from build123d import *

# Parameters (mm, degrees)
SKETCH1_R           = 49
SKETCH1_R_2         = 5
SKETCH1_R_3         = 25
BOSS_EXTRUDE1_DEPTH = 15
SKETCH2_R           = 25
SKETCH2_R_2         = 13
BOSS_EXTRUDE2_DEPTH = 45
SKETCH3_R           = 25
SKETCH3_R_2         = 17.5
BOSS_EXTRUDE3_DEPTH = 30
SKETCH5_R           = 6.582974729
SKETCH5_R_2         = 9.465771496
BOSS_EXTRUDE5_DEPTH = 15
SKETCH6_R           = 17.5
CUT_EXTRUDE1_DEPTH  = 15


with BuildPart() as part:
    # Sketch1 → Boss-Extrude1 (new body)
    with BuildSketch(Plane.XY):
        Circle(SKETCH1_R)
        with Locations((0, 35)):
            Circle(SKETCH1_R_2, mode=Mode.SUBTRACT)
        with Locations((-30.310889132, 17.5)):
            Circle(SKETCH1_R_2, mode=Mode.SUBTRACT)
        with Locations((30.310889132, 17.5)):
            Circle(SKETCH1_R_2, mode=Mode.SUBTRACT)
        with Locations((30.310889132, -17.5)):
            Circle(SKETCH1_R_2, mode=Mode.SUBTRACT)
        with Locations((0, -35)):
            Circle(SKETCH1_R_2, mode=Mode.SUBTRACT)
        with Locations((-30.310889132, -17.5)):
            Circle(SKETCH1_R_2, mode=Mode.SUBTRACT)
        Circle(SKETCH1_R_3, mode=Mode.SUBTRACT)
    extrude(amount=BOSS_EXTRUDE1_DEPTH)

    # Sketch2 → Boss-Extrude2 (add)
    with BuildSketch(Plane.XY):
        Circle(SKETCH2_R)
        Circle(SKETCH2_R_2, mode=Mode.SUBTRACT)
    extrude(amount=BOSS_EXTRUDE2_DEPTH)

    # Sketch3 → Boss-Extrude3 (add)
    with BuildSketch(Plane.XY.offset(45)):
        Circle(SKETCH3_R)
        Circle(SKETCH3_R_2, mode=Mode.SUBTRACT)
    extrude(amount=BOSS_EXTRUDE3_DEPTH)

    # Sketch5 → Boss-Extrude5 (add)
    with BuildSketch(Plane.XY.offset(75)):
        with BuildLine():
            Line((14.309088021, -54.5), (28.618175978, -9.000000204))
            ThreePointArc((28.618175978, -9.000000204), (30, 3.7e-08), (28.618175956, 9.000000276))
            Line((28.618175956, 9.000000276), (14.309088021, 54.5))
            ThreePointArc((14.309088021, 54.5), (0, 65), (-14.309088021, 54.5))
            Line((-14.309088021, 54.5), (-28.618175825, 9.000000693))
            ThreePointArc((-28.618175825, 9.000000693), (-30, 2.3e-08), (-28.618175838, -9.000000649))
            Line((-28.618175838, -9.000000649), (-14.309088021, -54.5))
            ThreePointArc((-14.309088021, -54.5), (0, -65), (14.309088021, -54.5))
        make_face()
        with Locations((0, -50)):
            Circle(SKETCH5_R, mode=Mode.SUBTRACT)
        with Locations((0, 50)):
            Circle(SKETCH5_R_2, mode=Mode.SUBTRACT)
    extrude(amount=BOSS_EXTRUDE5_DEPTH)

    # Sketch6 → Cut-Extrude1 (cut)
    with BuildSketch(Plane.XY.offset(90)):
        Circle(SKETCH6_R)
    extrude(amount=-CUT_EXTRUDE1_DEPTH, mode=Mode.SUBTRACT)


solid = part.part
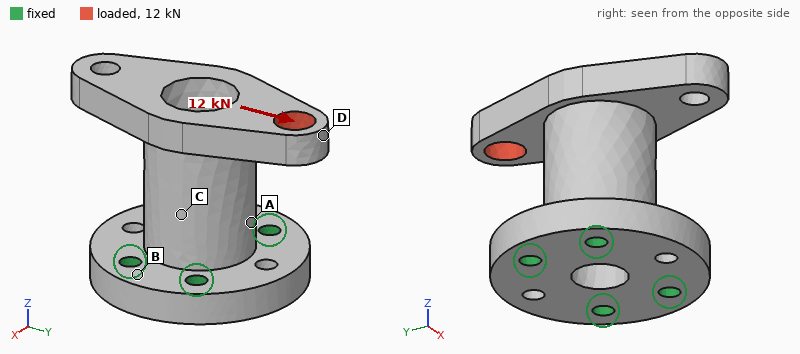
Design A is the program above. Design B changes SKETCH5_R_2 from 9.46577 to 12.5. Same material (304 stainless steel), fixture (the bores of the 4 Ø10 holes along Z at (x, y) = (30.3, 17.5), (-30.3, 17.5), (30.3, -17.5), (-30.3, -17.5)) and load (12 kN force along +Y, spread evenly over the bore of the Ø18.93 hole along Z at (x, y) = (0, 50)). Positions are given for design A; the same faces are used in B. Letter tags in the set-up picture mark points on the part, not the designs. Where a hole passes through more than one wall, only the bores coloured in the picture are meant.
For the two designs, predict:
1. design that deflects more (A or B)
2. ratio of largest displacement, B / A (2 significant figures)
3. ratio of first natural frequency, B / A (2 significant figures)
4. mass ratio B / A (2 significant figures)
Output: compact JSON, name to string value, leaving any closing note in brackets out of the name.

{"design that deflects more": "B", "ratio of largest displacement, B / A": "1.1", "ratio of first natural frequency, B / A": "1.0", "mass ratio B / A": "0.99"}
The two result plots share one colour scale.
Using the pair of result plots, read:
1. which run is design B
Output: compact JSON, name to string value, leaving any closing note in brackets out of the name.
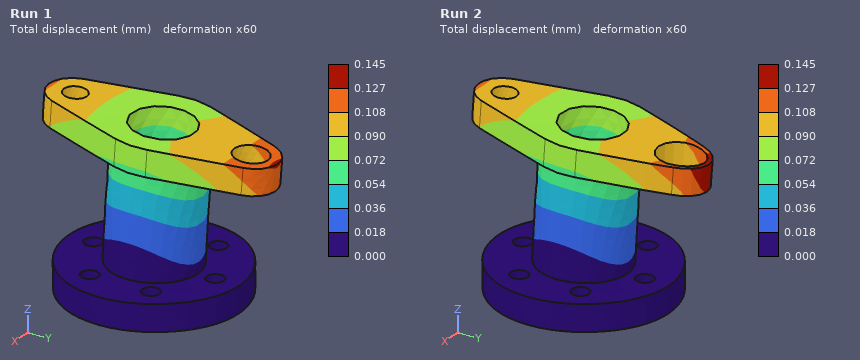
{"which run is design B": "Run 2"}
